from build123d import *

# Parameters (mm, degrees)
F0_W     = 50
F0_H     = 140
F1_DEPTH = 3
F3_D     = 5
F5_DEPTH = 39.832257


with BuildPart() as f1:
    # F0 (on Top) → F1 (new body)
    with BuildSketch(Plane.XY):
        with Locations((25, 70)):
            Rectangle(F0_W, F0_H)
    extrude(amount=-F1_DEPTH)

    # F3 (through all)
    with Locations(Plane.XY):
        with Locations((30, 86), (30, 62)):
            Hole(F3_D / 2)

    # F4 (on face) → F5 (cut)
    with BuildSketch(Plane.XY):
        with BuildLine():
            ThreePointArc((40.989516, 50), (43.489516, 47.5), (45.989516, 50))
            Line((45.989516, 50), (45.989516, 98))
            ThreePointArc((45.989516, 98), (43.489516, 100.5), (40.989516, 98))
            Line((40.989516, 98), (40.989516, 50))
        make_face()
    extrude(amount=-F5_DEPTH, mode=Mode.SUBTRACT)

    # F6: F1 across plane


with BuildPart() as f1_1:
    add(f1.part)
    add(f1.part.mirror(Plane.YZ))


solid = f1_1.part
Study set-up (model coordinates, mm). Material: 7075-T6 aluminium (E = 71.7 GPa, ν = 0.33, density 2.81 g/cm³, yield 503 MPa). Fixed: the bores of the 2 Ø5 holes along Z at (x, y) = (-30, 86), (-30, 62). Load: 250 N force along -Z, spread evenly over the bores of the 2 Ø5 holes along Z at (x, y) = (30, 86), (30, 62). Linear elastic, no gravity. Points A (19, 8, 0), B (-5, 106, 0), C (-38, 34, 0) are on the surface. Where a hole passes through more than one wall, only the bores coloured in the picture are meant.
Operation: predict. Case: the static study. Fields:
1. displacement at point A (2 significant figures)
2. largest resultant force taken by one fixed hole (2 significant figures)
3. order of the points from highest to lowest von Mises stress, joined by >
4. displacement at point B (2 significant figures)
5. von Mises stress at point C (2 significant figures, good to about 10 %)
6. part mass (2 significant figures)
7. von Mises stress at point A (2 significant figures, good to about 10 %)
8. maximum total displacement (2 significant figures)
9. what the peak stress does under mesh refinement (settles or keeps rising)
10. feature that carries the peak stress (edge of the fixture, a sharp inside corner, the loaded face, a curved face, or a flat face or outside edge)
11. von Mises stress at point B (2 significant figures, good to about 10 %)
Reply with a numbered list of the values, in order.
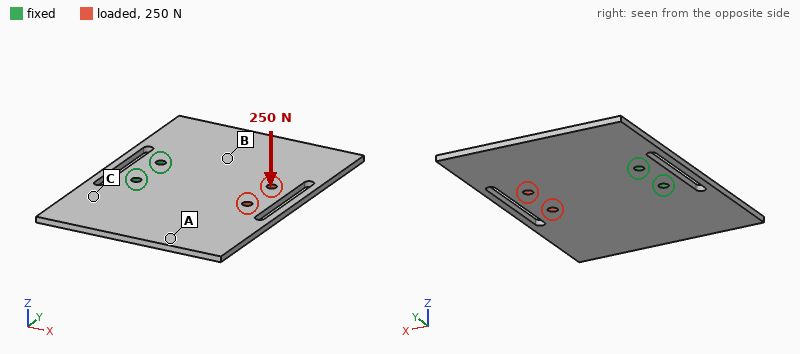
1. 0.77 mm
2. 130 N
3. B > C > A
4. 0.33 mm
5. 25 MPa
6. 110 g
7. 15 MPa
8. 1.8 mm
9. keeps rising
10. edge of the fixture
11. 44 MPa
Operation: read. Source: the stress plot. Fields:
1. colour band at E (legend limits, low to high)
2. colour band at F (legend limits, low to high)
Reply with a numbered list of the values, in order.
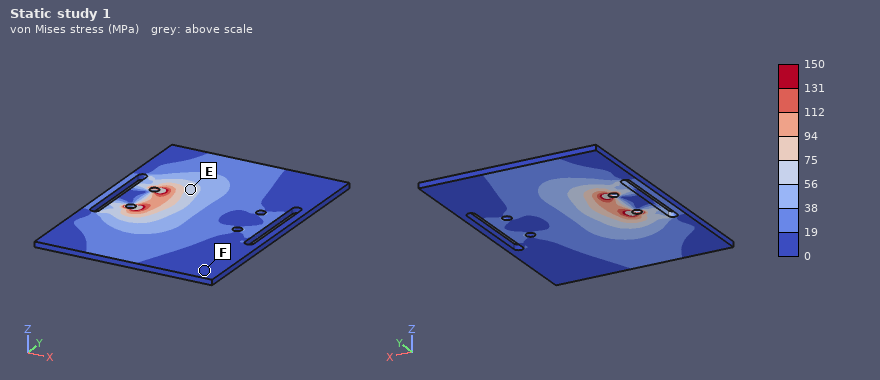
1. 56 to 75 MPa
2. 0 to 19 MPa
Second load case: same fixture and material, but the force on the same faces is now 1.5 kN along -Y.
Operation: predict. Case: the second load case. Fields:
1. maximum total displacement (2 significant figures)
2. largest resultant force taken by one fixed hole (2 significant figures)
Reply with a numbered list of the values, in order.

1. 0.15 mm
2. 3.3 kN
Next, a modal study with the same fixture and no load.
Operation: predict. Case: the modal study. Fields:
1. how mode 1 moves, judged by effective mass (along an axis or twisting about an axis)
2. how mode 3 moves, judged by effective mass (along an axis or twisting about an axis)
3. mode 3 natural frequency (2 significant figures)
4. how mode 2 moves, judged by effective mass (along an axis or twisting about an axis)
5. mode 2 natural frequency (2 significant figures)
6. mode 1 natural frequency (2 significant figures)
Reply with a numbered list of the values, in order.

1. along Z
2. along Z
3. 690 Hz
4. twisting about X
5. 380 Hz
6. 310 Hz
